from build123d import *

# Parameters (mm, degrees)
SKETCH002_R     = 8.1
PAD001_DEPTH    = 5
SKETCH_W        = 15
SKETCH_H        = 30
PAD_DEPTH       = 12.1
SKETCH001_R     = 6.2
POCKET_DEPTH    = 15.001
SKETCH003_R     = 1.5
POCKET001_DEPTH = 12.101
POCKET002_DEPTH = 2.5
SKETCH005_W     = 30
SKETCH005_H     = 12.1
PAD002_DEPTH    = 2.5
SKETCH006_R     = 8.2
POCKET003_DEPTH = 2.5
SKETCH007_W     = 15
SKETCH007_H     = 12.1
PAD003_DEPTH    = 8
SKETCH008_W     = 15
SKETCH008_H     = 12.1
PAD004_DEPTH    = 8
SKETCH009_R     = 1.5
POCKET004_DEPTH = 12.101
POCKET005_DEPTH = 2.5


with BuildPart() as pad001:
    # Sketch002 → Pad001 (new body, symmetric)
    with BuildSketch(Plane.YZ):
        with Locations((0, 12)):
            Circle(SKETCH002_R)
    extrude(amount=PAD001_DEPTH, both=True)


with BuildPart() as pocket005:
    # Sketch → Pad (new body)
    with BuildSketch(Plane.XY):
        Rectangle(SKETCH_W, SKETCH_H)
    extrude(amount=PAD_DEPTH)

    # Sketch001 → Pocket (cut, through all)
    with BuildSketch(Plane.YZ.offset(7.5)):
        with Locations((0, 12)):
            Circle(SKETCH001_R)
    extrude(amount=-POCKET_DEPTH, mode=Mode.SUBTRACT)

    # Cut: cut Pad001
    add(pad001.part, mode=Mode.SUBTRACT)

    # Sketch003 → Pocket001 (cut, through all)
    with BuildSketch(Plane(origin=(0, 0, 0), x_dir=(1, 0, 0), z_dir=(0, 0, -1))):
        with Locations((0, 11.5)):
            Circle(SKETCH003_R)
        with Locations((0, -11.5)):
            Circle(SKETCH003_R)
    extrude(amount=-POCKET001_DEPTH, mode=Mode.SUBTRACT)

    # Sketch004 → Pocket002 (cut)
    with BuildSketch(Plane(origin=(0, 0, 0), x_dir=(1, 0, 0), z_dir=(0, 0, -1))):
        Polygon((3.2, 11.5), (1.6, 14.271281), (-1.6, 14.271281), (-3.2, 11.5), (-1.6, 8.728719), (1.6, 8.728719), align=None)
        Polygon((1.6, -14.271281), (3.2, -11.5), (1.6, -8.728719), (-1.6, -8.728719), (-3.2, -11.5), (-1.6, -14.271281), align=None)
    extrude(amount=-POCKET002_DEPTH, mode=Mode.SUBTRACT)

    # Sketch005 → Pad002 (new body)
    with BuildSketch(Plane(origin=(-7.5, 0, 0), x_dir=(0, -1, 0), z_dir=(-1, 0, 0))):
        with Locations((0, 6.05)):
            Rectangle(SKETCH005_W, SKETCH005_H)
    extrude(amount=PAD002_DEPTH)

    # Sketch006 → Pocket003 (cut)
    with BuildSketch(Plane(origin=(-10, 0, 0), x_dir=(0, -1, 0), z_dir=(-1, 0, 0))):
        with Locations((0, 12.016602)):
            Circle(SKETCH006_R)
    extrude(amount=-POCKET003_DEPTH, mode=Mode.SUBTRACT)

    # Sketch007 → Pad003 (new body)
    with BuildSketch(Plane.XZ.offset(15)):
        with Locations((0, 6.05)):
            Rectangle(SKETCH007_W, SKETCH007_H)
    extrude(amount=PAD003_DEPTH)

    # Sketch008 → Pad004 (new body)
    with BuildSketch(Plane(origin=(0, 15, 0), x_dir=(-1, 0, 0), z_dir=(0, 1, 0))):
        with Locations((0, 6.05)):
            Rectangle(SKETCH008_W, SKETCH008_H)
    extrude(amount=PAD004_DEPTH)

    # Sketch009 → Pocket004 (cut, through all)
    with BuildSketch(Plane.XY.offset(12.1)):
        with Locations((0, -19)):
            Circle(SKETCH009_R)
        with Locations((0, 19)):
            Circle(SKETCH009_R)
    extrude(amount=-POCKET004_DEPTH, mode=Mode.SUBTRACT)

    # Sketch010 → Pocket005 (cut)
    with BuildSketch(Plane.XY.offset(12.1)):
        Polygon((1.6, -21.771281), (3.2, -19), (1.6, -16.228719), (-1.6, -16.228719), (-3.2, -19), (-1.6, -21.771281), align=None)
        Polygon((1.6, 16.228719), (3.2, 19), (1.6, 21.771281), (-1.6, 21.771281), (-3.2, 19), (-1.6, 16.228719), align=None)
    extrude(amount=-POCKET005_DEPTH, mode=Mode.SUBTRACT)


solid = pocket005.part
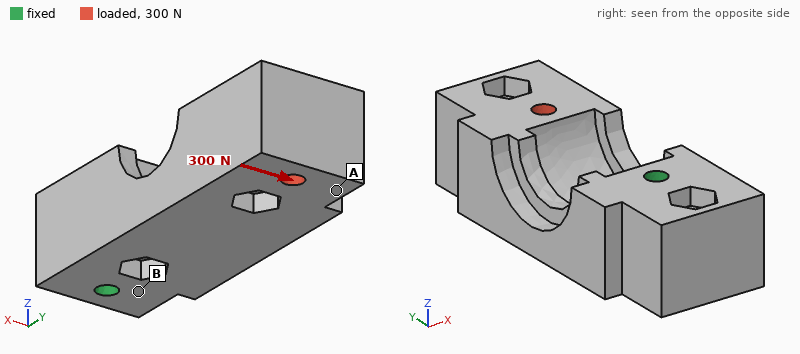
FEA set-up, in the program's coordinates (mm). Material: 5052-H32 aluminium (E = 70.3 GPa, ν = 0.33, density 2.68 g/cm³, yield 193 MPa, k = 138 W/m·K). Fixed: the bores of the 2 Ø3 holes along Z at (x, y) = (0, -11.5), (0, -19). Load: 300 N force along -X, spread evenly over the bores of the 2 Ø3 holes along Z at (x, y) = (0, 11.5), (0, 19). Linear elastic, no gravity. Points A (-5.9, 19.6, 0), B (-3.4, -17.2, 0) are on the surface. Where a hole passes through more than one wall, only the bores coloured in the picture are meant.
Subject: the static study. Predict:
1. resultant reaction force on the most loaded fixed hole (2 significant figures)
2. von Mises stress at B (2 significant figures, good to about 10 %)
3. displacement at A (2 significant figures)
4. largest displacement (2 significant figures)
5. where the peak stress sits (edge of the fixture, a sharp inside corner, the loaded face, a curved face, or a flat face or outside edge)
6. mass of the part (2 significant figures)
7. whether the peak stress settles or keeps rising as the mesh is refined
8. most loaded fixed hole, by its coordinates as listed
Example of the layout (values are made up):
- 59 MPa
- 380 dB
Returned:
- 990 N
- 12 MPa
- 26 µm
- 39 µm
- edge of the fixture
- 19 g
- keeps rising
- (0, -11.5)
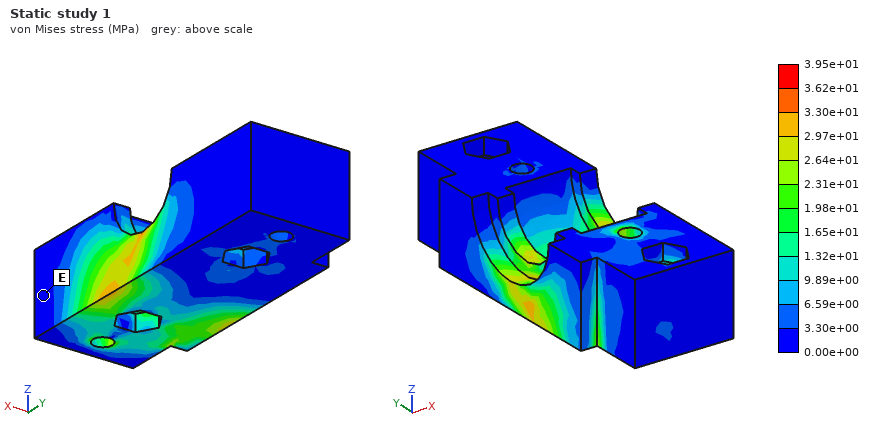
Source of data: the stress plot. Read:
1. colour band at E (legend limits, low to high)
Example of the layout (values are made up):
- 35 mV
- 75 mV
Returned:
- 0.00e+00 to 3.30e+00 MPa
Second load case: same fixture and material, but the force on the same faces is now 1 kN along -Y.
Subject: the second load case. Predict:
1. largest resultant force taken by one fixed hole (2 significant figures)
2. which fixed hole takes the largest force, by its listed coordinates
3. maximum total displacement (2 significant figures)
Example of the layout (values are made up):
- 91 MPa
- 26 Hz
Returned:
- 680 N
- (0, -11.5)
- 78 µm
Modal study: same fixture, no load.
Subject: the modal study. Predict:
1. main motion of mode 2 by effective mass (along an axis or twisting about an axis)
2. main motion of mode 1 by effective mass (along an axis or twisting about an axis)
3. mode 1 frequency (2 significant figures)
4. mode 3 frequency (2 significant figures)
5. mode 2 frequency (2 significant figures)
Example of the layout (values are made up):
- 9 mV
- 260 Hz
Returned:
- along X
- along Z
- 3300 Hz
- 11 kHz
- 5800 Hz
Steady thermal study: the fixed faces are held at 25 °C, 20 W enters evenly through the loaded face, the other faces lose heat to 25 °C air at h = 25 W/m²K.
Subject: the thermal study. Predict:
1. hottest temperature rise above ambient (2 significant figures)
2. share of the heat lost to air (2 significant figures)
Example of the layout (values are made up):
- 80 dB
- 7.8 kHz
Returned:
- 37 K
- 7.1 %
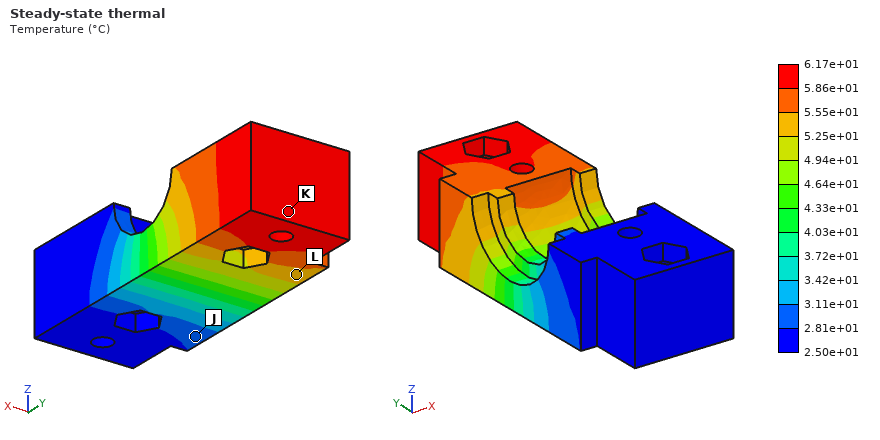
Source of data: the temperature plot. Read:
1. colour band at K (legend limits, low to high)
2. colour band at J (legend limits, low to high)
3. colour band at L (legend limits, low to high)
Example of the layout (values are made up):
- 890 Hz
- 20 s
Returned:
- 5.86e+01 to 6.17e+01 °C
- 2.81e+01 to 3.11e+01 °C
- 5.25e+01 to 5.55e+01 °C
